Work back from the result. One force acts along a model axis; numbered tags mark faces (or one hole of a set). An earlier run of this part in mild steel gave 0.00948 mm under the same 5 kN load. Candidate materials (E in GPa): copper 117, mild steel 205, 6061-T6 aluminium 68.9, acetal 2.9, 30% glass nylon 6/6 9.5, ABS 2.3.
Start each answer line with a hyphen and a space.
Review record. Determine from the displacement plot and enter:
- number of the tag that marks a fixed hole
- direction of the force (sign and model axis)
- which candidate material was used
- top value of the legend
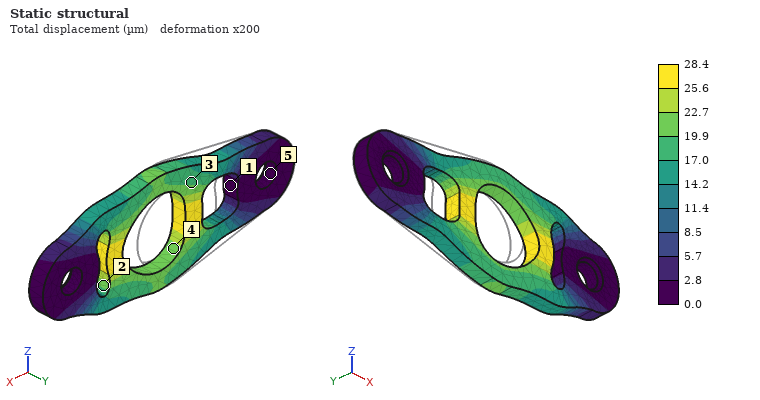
- 5
- +X
- 6061-T6 aluminium
- 28.4 µm
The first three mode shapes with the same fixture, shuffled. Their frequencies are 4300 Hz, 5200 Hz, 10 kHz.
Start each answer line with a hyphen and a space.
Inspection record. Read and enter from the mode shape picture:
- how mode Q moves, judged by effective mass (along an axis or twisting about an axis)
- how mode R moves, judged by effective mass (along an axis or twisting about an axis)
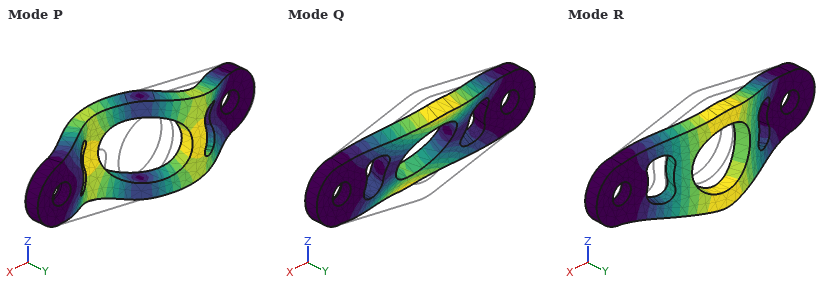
- twisting about X
- along Y
